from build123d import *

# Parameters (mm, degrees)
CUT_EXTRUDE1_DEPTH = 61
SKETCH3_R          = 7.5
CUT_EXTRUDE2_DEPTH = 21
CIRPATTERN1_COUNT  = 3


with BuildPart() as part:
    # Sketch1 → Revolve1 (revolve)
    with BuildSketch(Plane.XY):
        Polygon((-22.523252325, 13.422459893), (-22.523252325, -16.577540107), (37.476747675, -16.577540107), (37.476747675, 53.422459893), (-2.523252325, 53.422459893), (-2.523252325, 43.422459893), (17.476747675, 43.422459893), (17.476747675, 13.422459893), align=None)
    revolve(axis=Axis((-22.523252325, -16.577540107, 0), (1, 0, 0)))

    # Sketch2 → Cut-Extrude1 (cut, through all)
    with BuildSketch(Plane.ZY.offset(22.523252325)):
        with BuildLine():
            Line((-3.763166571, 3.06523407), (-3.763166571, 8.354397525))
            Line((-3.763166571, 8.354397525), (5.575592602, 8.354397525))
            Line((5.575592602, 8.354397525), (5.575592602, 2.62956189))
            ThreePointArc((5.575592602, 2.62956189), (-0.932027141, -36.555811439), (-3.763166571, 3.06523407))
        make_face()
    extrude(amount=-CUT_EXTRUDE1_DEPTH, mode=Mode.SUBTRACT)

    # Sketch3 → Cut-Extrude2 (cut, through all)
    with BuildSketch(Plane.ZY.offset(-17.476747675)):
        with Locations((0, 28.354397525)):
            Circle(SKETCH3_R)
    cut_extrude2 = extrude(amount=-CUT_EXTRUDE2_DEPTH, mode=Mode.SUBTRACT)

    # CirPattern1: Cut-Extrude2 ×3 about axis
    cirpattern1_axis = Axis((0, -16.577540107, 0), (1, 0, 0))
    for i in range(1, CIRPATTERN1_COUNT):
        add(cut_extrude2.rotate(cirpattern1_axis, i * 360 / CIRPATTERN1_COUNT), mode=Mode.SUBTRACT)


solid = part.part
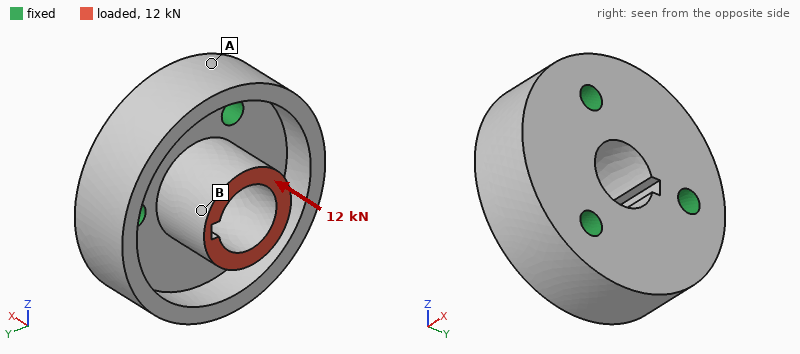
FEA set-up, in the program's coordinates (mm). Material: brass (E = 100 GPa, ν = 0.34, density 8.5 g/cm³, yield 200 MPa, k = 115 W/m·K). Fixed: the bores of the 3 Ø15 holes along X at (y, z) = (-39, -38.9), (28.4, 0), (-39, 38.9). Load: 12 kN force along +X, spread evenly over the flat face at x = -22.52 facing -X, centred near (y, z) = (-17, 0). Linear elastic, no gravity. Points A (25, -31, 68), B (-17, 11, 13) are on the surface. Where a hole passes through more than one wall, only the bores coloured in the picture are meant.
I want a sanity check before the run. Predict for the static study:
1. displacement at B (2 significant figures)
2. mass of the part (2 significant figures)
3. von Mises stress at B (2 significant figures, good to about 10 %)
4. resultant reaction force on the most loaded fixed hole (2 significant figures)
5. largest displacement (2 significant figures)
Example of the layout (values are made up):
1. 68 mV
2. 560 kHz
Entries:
1. 6.2 µm
2. 3.5 kg
3. 8.0 MPa
4. 4.2 kN
5. 6.8 µm
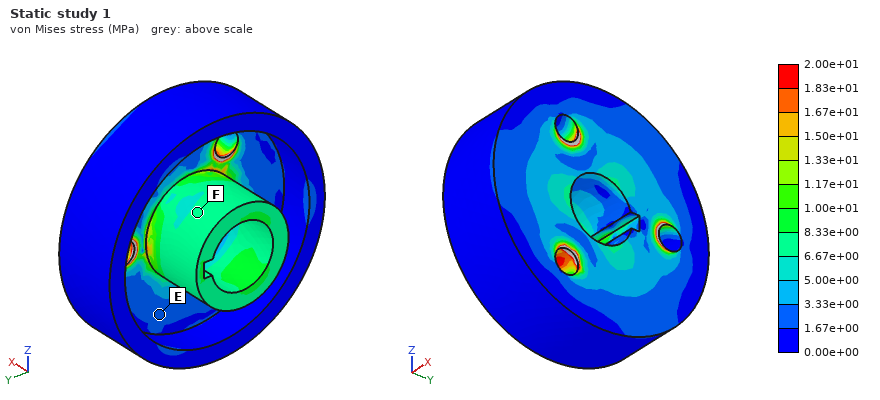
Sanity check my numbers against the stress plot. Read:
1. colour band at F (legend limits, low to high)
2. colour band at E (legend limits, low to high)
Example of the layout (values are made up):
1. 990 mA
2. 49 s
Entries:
1. 6.67e+00 to 8.33e+00 MPa
2. 1.67e+00 to 3.33e+00 MPa
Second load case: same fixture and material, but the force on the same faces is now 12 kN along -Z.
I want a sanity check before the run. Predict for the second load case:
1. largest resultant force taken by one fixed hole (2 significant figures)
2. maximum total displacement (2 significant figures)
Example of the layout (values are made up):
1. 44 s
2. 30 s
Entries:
1. 8.7 kN
2. 48 µm
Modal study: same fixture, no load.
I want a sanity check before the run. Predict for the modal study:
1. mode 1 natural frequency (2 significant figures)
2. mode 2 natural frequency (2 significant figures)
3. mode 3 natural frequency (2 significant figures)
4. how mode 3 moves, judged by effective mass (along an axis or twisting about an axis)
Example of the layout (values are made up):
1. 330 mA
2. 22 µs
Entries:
1. 3900 Hz
2. 3900 Hz
3. 5100 Hz
4. along X
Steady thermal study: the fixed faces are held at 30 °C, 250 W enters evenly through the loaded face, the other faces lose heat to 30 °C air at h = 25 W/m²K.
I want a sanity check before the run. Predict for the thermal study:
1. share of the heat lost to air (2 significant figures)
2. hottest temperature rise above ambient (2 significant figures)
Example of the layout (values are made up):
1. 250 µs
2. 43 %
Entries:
1. 8.4 %
2. 73 K
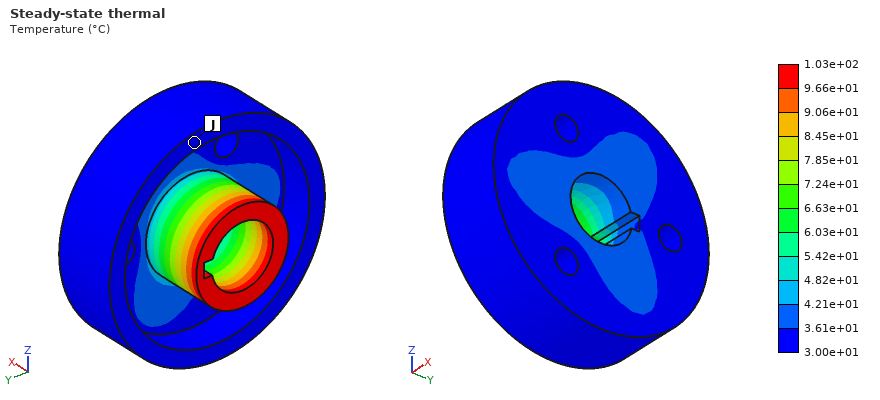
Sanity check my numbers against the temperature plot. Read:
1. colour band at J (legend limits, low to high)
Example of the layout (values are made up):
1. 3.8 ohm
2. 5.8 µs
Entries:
1. 3.00e+01 to 3.61e+01 °C
